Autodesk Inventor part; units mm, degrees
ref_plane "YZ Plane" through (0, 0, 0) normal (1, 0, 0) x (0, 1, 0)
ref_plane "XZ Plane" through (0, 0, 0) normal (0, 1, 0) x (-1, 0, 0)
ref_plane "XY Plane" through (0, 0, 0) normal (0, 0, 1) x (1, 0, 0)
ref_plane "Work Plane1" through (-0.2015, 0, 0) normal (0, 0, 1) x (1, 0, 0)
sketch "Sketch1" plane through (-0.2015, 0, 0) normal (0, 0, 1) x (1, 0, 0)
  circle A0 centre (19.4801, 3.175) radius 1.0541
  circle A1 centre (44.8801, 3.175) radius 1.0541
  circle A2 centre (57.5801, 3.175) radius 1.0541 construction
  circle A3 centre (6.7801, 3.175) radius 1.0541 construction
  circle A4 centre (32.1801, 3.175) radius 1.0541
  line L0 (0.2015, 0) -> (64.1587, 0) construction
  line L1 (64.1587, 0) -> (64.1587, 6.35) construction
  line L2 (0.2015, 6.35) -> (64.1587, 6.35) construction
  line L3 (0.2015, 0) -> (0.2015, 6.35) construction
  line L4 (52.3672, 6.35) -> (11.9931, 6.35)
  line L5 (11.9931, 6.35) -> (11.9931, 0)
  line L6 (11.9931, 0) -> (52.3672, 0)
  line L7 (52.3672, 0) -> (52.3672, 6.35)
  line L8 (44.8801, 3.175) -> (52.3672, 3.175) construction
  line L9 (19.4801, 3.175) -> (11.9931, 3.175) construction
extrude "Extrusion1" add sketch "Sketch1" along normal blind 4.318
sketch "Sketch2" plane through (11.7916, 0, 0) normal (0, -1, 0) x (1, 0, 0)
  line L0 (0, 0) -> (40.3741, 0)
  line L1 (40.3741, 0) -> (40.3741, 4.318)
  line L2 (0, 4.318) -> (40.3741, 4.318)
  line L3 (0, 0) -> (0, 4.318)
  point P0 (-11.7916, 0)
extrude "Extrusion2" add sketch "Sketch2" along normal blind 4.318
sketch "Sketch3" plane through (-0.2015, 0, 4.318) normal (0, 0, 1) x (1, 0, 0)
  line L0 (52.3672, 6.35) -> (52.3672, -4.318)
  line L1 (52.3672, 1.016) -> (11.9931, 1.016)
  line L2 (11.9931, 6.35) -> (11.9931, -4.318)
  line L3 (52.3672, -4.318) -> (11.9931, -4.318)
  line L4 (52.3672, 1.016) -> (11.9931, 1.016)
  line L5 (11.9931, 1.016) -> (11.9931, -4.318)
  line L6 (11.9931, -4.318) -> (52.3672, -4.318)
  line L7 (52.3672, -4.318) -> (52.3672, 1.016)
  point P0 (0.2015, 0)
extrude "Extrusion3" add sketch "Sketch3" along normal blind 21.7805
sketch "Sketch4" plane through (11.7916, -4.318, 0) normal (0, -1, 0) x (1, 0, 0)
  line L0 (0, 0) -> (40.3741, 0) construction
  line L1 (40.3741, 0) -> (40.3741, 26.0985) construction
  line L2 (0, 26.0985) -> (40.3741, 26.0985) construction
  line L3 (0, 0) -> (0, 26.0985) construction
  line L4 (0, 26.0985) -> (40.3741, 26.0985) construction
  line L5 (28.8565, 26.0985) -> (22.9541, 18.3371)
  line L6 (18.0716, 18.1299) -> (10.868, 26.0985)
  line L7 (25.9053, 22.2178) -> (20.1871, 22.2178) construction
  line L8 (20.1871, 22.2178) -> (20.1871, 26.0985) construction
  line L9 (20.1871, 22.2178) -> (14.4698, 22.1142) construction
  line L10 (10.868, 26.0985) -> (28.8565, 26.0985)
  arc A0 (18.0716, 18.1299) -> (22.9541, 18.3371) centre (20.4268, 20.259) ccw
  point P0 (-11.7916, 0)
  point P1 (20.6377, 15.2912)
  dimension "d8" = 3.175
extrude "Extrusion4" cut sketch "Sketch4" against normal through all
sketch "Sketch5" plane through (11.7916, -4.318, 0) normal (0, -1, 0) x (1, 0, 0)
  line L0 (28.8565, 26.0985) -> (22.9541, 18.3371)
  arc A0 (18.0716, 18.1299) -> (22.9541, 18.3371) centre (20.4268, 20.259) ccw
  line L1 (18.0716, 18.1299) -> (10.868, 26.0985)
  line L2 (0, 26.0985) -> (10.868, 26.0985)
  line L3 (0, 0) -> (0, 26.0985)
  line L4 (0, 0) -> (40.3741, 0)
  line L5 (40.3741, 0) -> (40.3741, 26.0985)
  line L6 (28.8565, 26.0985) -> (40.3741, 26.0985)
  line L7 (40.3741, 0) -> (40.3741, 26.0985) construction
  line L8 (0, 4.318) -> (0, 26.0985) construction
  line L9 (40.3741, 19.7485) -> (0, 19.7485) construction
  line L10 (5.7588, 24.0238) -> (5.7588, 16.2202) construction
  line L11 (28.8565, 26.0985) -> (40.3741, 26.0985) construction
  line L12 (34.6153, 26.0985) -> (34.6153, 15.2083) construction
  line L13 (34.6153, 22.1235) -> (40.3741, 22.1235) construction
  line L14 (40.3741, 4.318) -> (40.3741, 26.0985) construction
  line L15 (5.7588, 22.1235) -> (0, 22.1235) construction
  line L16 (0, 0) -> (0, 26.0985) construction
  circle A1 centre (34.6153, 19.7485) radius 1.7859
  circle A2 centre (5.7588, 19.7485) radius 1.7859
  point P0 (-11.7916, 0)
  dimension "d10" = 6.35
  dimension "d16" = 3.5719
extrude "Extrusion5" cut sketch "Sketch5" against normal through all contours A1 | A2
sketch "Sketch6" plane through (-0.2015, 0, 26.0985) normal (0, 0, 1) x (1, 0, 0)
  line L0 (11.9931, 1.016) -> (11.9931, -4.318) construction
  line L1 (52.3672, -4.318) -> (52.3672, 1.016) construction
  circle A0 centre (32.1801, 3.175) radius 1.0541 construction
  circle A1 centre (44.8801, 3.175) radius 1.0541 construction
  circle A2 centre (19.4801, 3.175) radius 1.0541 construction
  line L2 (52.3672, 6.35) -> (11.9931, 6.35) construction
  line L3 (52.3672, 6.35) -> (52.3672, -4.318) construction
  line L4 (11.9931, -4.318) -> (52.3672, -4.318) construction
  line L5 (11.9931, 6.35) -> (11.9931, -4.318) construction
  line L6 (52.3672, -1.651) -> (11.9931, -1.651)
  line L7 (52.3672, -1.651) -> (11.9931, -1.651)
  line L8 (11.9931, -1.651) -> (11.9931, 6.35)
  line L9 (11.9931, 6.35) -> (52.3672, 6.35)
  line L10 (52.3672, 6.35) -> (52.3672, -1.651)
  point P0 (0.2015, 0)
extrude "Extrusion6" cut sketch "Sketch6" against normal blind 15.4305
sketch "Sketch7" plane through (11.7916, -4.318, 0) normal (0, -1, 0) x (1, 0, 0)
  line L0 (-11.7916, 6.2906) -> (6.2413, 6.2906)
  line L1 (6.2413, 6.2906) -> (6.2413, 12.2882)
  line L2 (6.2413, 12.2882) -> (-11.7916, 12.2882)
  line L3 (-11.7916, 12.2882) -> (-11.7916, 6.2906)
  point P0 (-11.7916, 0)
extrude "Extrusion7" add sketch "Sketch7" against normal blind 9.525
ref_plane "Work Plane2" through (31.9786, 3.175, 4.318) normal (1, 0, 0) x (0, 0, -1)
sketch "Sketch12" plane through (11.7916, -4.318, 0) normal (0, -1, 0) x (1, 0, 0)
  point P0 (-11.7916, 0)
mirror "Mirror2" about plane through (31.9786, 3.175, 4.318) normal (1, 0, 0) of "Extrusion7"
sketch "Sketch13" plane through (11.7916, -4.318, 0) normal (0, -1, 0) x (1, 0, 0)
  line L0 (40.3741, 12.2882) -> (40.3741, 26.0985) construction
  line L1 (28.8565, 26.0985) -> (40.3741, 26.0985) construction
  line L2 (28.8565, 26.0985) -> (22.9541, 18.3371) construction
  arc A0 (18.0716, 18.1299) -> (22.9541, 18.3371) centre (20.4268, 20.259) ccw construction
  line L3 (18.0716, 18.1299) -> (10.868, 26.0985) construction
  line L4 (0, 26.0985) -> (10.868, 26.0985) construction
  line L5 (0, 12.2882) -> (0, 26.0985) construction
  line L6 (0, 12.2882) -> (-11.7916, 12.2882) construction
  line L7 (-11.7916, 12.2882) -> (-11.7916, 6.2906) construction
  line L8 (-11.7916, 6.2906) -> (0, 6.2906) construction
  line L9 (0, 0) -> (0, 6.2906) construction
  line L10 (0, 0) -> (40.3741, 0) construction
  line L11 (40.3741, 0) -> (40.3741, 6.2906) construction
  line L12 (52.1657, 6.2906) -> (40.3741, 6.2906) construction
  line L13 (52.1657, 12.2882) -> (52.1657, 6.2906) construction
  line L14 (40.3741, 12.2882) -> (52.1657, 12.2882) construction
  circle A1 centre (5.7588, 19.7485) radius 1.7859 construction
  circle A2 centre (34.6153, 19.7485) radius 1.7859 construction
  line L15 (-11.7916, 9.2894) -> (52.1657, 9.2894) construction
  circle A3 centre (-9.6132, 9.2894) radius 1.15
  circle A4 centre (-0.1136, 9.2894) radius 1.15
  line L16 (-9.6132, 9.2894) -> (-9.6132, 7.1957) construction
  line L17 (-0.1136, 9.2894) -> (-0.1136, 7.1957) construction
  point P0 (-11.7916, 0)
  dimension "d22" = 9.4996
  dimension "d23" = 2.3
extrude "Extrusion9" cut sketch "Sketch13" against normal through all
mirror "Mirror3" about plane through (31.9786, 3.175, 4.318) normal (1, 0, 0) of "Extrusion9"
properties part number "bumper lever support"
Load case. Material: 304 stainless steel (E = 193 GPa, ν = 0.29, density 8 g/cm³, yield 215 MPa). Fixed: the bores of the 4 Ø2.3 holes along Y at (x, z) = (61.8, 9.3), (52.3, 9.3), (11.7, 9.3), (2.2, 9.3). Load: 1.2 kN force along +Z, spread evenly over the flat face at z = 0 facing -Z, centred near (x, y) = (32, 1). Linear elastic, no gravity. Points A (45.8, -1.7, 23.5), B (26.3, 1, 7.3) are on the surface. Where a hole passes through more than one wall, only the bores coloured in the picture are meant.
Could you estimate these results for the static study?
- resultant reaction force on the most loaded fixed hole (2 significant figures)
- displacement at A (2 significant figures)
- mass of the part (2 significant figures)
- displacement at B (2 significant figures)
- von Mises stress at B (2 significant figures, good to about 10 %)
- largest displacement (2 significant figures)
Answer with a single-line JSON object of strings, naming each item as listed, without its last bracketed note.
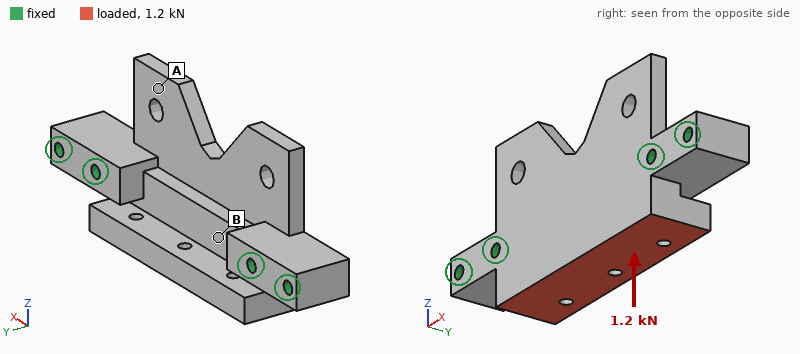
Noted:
{"resultant reaction force on the most loaded fixed hole": "680 N", "displacement at A": "3.1 µm", "mass of the part": "49 g", "displacement at B": "3.5 µm", "von Mises stress at B": "12 MPa", "largest displacement": "8.2 µm"}
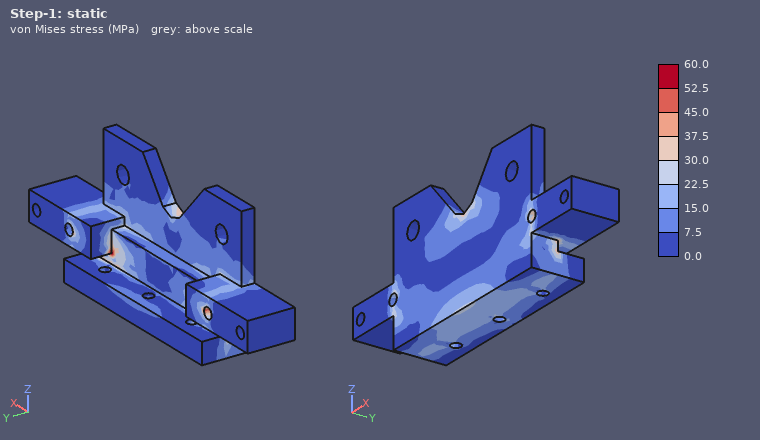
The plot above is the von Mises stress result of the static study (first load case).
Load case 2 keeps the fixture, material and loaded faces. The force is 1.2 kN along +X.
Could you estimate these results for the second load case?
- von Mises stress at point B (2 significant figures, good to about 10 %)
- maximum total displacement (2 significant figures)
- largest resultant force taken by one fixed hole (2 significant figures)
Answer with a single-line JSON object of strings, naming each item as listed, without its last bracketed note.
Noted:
{"von Mises stress at point B": "8.4 MPa", "maximum total displacement": "1.8 µm", "largest resultant force taken by one fixed hole": "620 N"}
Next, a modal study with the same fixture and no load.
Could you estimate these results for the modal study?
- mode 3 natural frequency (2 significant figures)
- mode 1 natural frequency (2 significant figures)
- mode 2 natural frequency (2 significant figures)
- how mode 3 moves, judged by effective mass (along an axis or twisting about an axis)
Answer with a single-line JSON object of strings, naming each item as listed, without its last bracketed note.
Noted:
{"mode 3 natural frequency": "15 kHz", "mode 1 natural frequency": "8500 Hz", "mode 2 natural frequency": "10 kHz", "how mode 3 moves, judged by effective mass": "along Y"}
